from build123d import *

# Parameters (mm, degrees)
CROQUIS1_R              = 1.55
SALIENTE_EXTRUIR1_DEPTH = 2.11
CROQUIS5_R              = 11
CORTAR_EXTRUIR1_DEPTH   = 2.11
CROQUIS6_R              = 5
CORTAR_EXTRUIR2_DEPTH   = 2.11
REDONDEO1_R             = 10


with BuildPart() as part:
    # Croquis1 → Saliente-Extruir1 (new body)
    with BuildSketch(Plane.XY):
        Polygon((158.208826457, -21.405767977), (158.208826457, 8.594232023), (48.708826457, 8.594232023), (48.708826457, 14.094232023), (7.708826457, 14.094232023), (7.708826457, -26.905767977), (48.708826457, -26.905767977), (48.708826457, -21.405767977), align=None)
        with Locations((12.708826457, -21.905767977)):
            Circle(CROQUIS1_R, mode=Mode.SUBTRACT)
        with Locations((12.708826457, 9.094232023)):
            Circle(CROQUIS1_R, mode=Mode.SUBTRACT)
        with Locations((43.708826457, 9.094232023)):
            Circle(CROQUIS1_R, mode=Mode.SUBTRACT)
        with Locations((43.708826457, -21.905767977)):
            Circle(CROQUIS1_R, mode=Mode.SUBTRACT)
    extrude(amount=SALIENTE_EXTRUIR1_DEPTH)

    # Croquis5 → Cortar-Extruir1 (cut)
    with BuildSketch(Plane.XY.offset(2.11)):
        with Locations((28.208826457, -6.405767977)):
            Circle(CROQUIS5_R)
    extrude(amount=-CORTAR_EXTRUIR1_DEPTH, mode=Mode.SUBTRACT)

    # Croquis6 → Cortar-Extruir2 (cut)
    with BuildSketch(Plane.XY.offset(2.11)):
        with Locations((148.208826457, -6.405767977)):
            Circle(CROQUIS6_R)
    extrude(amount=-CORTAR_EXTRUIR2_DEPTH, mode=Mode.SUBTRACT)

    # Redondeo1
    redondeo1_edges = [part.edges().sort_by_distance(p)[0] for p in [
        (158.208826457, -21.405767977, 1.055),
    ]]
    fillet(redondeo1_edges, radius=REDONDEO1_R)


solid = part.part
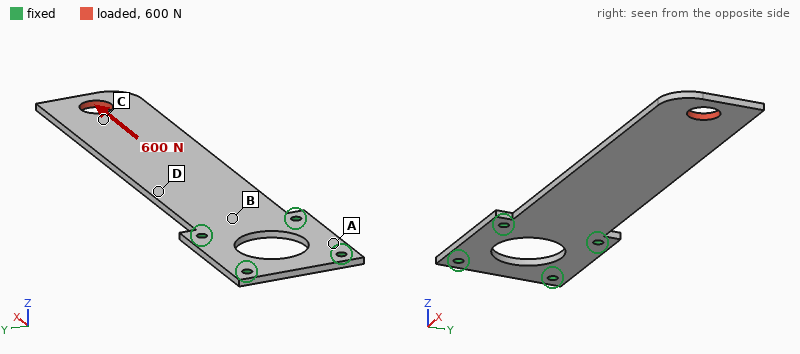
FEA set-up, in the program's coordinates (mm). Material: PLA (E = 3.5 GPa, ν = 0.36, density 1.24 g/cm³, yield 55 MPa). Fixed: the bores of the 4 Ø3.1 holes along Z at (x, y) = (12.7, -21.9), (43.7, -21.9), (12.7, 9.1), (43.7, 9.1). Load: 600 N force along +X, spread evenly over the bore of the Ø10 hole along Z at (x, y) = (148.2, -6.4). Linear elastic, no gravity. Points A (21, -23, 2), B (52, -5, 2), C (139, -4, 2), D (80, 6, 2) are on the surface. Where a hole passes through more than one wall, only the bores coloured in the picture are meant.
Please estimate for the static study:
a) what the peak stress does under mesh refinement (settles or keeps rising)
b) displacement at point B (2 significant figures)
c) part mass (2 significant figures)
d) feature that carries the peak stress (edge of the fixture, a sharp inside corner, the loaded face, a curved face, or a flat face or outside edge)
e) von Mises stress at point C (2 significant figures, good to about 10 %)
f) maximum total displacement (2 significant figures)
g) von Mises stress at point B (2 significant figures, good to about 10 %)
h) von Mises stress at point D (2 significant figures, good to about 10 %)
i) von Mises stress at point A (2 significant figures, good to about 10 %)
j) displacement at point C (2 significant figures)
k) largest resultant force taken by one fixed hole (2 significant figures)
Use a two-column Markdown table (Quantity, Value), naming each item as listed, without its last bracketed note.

| Quantity | Value |
|---|---|
| what the peak stress does under mesh refinement | keeps rising |
| displacement at point B | 0.067 mm |
| part mass | 12 g |
| feature that carries the peak stress | edge of the fixture |
| von Mises stress at point C | 11 MPa |
| maximum total displacement | 0.39 mm |
| von Mises stress at point B | 4.8 MPa |
| von Mises stress at point D | 9.4 MPa |
| von Mises stress at point A | 2.3 MPa |
| displacement at point C | 0.29 mm |
| largest resultant force taken by one fixed hole | 290 N |
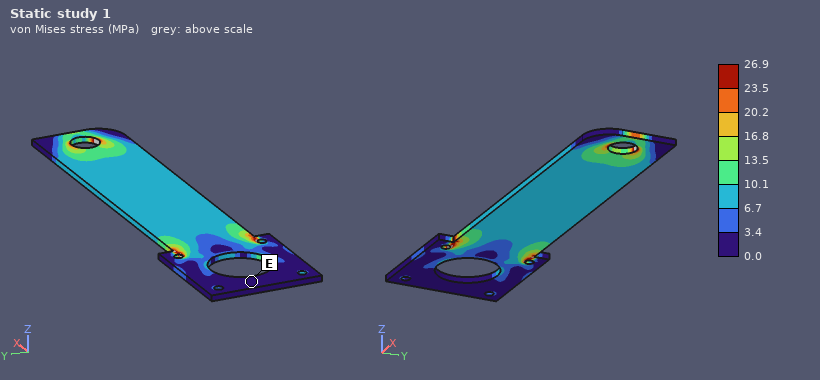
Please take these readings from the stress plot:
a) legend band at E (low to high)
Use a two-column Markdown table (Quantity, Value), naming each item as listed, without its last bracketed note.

| Quantity | Value |
|---|---|
| legend band at E | 0.0 to 3.4 MPa |
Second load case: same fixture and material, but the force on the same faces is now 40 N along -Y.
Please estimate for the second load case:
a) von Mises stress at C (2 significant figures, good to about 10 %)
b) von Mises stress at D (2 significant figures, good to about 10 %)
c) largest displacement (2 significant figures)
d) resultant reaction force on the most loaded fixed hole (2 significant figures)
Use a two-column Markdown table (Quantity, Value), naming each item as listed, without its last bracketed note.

| Quantity | Value |
|---|---|
| von Mises stress at C | 2.0 MPa |
| von Mises stress at D | 7.0 MPa |
| largest displacement | 1.1 mm |
| resultant reaction force on the most loaded fixed hole | 140 N |
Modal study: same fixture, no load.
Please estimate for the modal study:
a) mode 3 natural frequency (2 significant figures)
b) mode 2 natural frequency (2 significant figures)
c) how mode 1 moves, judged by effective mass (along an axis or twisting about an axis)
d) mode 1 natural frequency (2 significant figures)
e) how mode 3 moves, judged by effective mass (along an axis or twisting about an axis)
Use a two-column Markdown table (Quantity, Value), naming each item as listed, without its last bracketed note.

| Quantity | Value |
|---|---|
| mode 3 natural frequency | 340 Hz |
| mode 2 natural frequency | 280 Hz |
| how mode 1 moves, judged by effective mass | along Z |
| mode 1 natural frequency | 45 Hz |
| how mode 3 moves, judged by effective mass | twisting about X |
